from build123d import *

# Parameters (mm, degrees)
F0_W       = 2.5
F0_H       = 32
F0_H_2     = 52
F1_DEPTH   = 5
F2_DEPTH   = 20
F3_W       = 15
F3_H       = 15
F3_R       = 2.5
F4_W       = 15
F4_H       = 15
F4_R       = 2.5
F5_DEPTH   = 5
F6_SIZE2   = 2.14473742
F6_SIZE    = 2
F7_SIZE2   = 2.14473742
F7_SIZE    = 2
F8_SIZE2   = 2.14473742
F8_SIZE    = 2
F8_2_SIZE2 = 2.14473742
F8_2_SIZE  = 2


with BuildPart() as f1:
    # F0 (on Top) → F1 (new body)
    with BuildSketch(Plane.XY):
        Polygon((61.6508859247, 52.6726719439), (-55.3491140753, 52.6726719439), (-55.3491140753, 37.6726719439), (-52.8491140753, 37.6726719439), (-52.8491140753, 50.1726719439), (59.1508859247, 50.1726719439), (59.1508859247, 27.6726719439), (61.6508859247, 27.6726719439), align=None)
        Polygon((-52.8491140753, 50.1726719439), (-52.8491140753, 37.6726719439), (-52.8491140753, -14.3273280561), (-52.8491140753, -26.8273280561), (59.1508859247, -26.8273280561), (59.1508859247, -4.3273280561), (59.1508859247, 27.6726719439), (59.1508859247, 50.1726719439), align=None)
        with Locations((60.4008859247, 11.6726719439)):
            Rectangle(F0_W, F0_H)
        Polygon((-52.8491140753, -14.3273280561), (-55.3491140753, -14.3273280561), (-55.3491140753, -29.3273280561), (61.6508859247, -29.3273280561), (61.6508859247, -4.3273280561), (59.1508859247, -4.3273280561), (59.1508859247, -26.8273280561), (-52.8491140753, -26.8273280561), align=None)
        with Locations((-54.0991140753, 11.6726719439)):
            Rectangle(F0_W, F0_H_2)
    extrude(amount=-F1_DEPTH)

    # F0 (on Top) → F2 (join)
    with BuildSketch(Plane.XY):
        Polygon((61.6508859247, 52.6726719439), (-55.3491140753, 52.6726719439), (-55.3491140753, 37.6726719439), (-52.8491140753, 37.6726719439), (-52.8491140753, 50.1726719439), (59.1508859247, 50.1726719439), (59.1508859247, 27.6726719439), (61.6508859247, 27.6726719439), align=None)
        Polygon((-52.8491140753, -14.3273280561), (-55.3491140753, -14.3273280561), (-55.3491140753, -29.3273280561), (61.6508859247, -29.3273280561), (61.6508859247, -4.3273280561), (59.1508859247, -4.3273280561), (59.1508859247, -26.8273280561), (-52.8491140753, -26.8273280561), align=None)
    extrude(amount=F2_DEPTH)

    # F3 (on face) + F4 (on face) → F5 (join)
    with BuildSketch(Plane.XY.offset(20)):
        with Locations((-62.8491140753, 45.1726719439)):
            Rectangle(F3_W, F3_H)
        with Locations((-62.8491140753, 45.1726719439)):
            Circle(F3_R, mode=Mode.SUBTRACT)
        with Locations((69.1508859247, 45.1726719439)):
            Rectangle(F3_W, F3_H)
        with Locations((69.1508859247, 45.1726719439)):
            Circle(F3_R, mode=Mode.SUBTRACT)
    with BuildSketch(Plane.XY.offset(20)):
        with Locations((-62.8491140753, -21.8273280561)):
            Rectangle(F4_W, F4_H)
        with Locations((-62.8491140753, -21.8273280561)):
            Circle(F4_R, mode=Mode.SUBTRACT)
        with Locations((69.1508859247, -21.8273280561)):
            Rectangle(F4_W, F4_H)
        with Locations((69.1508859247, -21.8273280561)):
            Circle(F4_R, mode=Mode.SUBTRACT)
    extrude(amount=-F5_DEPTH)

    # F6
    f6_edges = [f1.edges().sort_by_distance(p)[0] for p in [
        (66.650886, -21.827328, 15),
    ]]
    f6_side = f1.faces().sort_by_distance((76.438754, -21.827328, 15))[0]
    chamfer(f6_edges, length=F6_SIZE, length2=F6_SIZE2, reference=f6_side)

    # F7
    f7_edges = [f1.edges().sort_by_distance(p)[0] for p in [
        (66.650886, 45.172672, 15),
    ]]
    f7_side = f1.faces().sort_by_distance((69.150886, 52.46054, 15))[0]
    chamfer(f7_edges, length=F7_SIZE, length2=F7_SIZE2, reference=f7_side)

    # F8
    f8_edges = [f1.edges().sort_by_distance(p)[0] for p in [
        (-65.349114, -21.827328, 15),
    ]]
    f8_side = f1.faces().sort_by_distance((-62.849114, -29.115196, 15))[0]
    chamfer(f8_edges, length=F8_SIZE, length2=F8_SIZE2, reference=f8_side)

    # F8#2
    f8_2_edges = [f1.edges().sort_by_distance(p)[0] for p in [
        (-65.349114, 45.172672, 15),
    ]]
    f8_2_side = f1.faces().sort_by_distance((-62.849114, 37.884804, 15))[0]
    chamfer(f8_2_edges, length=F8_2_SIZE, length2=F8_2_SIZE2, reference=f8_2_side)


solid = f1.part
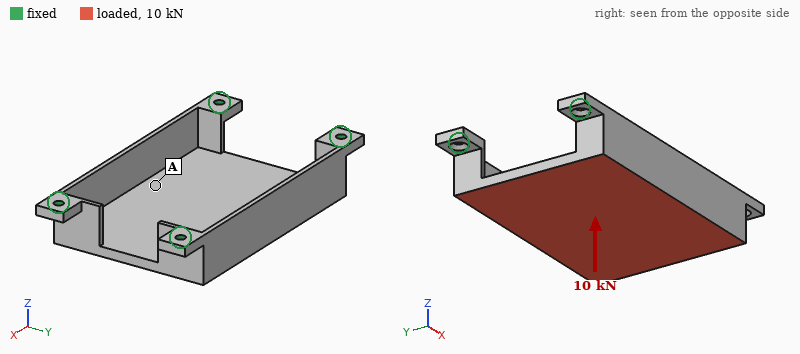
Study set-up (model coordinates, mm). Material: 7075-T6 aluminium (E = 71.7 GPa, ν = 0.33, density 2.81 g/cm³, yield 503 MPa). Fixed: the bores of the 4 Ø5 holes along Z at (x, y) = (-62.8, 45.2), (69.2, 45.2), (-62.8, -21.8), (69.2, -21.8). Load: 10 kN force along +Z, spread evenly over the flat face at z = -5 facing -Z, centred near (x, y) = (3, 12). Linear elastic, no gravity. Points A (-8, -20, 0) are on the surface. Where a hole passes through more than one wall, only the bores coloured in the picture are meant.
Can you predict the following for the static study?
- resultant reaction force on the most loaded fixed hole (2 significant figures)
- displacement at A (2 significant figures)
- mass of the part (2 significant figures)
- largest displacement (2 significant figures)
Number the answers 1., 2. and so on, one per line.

1. 3.3 kN
2. 0.26 mm
3. 190 g
4. 0.49 mm
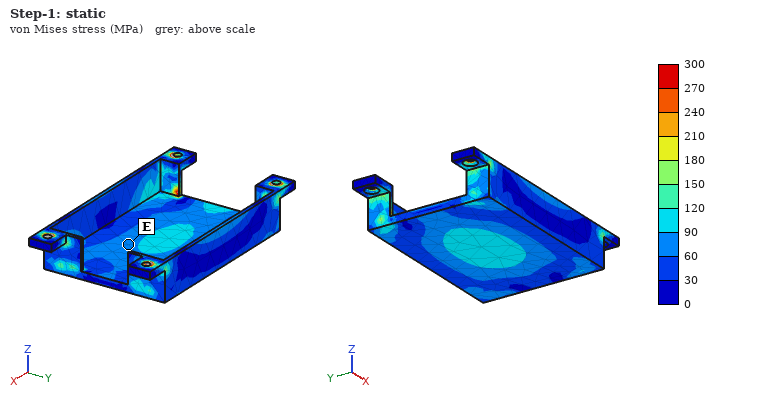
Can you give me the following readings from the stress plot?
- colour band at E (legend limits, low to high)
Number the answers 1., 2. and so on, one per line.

1. 60 to 90 MPa
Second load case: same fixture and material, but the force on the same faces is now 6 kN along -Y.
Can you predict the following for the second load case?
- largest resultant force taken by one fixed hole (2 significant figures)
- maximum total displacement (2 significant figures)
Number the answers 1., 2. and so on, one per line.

1. 2.1 kN
2. 0.24 mm
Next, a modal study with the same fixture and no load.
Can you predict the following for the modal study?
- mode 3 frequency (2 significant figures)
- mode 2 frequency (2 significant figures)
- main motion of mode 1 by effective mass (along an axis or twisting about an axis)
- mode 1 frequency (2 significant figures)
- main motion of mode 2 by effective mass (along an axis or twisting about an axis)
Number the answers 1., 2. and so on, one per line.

1. 4100 Hz
2. 2300 Hz
3. along Y
4. 2200 Hz
5. along Z
